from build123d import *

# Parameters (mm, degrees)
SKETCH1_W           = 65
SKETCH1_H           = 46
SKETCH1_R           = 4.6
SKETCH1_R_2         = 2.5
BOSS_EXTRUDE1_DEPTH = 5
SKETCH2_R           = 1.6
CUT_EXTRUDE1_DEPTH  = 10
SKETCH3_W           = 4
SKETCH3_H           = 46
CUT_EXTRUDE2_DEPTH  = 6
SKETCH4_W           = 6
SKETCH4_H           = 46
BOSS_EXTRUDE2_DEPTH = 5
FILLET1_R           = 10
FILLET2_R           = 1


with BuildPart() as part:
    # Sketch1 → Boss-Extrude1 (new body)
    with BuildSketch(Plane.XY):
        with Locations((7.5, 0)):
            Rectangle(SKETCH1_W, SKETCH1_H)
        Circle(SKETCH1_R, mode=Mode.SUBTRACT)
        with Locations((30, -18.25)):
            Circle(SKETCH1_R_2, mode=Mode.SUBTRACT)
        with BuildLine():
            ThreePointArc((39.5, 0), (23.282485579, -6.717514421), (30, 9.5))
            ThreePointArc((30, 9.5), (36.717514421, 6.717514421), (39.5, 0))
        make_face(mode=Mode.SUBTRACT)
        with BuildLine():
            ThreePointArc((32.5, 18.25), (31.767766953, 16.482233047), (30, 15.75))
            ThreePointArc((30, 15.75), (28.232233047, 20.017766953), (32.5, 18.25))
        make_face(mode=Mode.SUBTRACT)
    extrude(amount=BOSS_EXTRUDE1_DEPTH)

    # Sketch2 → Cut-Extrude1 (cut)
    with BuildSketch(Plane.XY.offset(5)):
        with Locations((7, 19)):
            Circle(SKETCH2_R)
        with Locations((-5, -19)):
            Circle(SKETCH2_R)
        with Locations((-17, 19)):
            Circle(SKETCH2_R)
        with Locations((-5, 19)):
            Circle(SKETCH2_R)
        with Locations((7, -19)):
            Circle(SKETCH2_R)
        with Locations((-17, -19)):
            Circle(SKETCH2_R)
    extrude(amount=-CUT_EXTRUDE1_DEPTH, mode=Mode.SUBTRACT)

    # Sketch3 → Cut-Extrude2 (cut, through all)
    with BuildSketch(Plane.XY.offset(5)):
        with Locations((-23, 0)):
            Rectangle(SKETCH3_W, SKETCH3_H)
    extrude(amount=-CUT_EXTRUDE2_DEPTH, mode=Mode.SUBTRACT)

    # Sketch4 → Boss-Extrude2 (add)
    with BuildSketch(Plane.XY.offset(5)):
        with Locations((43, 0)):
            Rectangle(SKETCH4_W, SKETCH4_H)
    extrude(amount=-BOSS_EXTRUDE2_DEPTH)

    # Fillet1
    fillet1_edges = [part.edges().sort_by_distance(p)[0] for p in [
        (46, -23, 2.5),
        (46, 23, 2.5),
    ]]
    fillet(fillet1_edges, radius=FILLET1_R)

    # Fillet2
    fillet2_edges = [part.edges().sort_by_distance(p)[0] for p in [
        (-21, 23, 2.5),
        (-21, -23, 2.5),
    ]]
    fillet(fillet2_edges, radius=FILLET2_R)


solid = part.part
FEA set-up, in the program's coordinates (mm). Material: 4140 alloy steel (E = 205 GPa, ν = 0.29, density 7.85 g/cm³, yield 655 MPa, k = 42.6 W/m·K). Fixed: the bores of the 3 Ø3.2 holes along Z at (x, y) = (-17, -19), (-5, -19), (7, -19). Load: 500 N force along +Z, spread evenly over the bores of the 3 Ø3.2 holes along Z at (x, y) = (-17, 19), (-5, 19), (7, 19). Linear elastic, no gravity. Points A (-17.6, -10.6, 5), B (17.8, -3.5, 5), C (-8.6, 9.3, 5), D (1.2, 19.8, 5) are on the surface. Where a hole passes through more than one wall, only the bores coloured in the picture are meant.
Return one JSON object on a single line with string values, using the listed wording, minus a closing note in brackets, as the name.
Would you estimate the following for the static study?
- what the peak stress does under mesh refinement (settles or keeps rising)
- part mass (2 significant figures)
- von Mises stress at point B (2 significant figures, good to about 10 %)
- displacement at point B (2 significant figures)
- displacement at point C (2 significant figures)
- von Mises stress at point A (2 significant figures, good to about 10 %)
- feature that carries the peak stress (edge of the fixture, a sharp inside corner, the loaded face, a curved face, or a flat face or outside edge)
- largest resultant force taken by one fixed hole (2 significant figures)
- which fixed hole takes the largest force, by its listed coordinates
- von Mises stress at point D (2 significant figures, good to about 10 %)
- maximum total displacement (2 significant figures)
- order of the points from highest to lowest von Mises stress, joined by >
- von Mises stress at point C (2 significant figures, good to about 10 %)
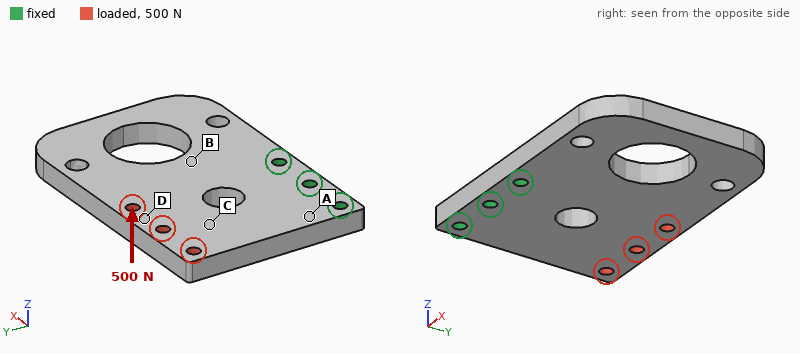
{"what the peak stress does under mesh refinement": "keeps rising", "part mass": "100 g", "von Mises stress at point B": "54 MPa", "displacement at point B": "0.024 mm", "displacement at point C": "0.071 mm", "von Mises stress at point A": "96 MPa", "feature that carries the peak stress": "edge of the fixture", "largest resultant force taken by one fixed hole": "270 N", "which fixed hole takes the largest force, by its listed coordinates": "(-5, -19)", "von Mises stress at point D": "16 MPa", "maximum total displacement": "0.13 mm", "order of the points from highest to lowest von Mises stress, joined by >": "A > B > C > D", "von Mises stress at point C": "27 MPa"}
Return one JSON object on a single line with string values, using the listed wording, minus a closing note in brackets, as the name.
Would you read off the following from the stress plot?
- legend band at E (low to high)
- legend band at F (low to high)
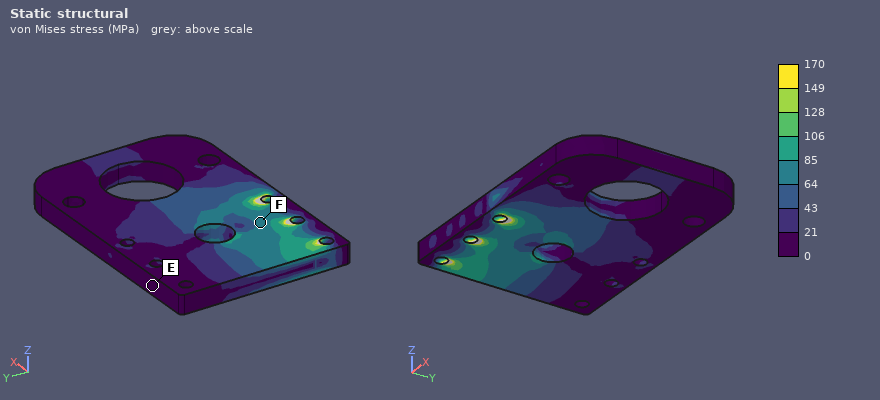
{"legend band at E": "0 to 21 MPa", "legend band at F": "64 to 85 MPa"}
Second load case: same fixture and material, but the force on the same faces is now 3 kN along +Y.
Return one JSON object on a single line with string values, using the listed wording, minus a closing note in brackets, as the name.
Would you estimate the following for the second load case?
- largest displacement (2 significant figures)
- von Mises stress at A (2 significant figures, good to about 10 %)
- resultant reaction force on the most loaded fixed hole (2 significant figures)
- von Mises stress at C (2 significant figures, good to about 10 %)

{"largest displacement": "4.7 µm", "von Mises stress at A": "23 MPa", "resultant reaction force on the most loaded fixed hole": "1.1 kN", "von Mises stress at C": "22 MPa"}
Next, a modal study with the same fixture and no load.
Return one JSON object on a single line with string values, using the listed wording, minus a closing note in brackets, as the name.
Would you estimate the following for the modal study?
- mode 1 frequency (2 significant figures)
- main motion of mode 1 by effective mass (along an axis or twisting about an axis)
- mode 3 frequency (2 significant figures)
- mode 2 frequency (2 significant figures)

{"mode 1 frequency": "1600 Hz", "main motion of mode 1 by effective mass": "along Z", "mode 3 frequency": "4800 Hz", "mode 2 frequency": "2600 Hz"}
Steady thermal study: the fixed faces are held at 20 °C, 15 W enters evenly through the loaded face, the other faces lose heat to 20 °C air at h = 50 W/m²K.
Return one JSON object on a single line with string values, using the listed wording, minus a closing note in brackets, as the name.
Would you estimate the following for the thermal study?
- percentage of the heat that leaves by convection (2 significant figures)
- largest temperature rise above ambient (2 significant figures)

{"percentage of the heat that leaves by convection": "45 %", "largest temperature rise above ambient": "60 K"}
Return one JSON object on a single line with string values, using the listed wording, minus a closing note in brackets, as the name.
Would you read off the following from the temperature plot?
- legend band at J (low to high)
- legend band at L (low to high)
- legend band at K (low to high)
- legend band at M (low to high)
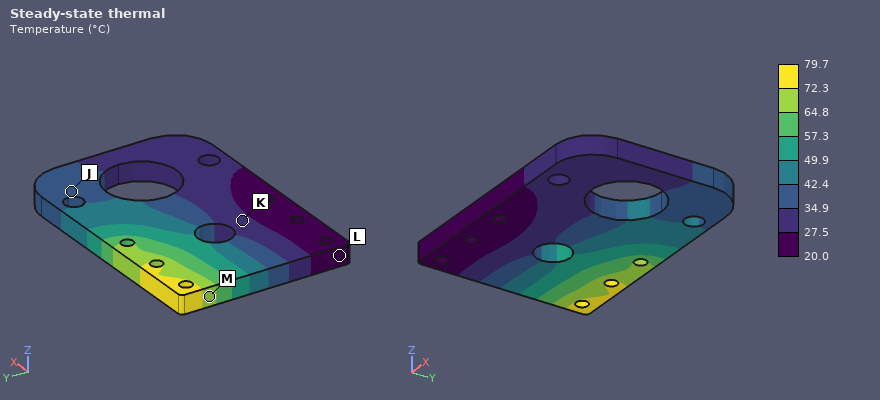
{"legend band at J": "34.9 to 42.4 °C", "legend band at L": "20.0 to 27.5 °C", "legend band at K": "27.5 to 34.9 °C", "legend band at M": "64.8 to 72.3 °C"}
